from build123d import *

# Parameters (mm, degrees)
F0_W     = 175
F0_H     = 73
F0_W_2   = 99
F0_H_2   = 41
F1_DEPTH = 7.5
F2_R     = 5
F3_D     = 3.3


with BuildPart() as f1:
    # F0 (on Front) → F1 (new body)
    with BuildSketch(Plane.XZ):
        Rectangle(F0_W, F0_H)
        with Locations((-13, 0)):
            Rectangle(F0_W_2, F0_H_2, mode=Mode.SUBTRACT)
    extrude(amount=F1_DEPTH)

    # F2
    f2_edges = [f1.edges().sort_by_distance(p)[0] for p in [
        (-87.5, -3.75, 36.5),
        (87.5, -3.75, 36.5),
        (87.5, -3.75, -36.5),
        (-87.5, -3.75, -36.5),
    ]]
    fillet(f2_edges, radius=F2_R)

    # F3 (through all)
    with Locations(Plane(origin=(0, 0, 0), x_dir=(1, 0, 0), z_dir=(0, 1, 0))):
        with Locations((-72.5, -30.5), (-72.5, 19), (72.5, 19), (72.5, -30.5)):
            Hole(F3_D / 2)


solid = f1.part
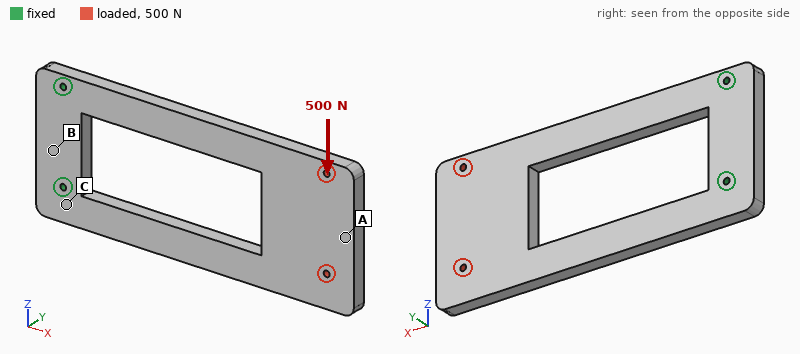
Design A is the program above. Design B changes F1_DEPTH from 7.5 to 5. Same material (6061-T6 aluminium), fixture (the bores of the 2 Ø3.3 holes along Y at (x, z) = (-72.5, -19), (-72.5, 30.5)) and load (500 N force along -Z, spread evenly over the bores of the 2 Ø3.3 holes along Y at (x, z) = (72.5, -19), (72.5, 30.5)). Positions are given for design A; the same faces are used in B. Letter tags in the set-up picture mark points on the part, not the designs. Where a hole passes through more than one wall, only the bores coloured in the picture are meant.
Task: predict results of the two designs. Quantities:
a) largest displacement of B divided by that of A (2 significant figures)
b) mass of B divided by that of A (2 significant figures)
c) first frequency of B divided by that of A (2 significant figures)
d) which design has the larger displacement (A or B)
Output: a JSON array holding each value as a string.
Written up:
["1.5", "0.67", "0.67", "B"]
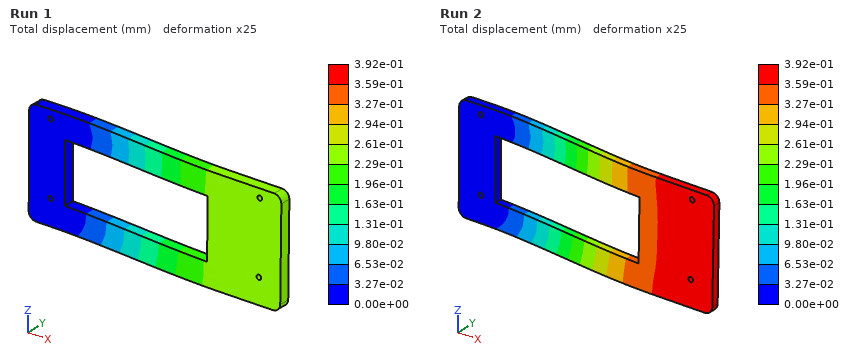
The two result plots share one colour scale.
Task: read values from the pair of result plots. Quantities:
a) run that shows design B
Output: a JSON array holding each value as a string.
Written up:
["Run 2"]
